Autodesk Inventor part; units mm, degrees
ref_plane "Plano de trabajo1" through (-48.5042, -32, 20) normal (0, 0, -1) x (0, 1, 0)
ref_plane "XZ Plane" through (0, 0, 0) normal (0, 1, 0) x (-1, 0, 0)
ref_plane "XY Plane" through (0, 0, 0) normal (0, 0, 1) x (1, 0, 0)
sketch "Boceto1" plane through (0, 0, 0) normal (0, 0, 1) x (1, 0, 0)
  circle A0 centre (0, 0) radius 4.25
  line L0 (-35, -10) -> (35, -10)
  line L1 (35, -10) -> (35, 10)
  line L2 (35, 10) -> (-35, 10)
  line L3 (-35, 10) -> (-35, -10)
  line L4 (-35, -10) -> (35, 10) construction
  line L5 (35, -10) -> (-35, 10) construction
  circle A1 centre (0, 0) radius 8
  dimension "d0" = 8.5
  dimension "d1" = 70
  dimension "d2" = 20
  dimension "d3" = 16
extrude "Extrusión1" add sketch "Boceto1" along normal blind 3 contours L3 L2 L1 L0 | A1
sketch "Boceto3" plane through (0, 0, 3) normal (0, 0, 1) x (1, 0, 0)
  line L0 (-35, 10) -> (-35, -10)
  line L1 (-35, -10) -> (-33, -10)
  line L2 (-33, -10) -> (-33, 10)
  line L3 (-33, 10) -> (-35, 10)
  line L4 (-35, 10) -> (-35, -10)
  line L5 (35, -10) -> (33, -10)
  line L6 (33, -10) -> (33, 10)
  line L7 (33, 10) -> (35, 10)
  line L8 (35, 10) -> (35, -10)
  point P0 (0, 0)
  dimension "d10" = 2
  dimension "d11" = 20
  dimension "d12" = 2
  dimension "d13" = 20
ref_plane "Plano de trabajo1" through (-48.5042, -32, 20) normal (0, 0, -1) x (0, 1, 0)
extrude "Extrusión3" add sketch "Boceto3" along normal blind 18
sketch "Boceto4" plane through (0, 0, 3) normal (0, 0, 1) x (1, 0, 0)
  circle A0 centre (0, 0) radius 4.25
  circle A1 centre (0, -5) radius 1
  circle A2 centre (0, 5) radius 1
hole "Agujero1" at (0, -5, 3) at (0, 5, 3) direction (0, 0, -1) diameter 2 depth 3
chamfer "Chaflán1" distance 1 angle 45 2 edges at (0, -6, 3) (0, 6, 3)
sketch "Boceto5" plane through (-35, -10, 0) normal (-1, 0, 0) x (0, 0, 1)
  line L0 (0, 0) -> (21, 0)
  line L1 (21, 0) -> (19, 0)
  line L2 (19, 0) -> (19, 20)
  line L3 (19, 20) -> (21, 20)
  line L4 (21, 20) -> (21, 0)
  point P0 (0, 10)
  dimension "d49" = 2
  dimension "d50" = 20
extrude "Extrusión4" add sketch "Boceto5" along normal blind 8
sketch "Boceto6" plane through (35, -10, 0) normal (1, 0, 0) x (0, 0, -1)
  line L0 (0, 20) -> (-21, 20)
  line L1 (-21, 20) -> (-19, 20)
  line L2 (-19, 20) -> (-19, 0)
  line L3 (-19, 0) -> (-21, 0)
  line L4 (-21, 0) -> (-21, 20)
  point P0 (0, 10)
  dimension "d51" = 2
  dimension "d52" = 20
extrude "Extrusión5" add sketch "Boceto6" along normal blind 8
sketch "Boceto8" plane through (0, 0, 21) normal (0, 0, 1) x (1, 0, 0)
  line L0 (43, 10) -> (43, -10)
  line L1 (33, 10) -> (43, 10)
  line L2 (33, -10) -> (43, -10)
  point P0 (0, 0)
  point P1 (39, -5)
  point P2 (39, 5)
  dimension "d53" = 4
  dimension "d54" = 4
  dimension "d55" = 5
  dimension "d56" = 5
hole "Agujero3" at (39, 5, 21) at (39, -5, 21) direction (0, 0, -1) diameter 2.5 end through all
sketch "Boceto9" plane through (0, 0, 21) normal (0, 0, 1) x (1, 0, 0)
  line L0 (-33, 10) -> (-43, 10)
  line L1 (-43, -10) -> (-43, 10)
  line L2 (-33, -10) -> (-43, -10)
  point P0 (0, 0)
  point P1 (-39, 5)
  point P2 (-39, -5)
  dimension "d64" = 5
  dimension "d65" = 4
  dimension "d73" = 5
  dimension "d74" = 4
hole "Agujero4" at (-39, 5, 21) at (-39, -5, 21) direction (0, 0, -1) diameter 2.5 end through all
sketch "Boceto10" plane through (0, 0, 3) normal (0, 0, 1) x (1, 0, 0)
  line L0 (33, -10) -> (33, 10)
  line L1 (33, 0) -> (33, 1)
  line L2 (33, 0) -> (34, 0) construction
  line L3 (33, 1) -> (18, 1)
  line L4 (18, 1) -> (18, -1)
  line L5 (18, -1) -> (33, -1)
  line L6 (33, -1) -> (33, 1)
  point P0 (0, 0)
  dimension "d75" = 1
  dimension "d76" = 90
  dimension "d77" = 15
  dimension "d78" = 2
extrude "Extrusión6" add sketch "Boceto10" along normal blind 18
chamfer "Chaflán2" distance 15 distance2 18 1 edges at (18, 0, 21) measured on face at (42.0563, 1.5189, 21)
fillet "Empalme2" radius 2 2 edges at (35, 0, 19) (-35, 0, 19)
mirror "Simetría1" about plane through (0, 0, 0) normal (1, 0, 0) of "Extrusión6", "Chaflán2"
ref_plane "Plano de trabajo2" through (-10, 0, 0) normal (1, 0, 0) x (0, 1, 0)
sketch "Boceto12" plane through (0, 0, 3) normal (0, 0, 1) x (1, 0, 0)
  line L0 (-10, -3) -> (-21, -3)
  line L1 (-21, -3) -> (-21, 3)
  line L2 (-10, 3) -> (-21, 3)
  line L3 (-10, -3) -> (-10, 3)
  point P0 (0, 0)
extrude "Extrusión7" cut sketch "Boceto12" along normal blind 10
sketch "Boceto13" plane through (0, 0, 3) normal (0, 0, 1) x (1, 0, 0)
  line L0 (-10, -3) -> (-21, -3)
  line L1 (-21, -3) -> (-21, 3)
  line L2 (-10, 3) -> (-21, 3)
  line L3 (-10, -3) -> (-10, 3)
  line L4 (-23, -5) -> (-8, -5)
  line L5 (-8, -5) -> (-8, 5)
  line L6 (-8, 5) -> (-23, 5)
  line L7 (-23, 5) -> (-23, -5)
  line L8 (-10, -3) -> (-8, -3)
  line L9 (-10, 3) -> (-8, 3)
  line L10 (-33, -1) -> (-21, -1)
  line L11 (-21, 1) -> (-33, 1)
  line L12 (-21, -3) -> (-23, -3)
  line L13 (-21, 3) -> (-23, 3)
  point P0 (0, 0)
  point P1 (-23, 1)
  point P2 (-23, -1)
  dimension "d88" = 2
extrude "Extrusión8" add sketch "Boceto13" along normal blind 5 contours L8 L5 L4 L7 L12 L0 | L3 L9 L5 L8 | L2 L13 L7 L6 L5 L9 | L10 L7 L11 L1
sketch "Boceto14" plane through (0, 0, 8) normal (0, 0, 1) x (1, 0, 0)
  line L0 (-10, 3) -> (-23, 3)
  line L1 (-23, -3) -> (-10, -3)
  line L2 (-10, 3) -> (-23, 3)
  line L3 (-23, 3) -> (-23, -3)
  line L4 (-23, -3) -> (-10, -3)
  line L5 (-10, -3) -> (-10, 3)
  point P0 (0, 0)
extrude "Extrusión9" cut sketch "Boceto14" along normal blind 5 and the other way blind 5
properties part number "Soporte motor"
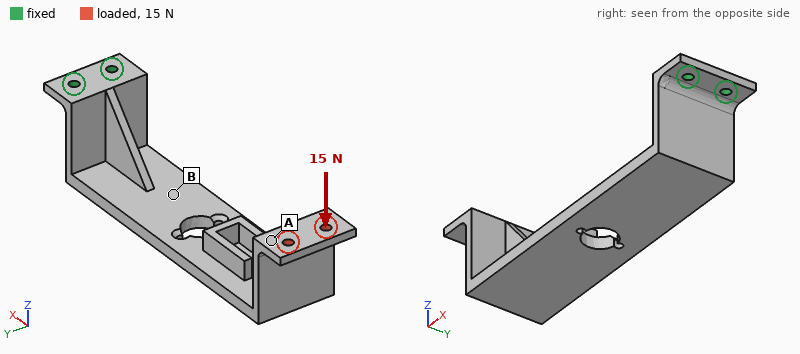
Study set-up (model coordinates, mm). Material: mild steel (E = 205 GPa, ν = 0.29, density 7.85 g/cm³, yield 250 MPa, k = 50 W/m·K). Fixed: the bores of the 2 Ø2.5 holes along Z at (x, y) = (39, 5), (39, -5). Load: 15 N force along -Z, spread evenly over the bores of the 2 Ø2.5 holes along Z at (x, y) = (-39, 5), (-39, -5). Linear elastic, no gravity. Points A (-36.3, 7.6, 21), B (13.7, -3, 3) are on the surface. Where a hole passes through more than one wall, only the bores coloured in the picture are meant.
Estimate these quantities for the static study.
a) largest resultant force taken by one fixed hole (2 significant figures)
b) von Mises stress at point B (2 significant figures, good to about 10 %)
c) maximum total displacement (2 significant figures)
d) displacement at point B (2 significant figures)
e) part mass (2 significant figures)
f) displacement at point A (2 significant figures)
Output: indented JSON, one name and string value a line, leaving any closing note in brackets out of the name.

{
  "largest resultant force taken by one fixed hole": "13 N",
  "von Mises stress at point B": "25 MPa",
  "maximum total displacement": "0.36 mm",
  "displacement at point B": "0.069 mm",
  "part mass": "55 g",
  "displacement at point A": "0.33 mm"
}
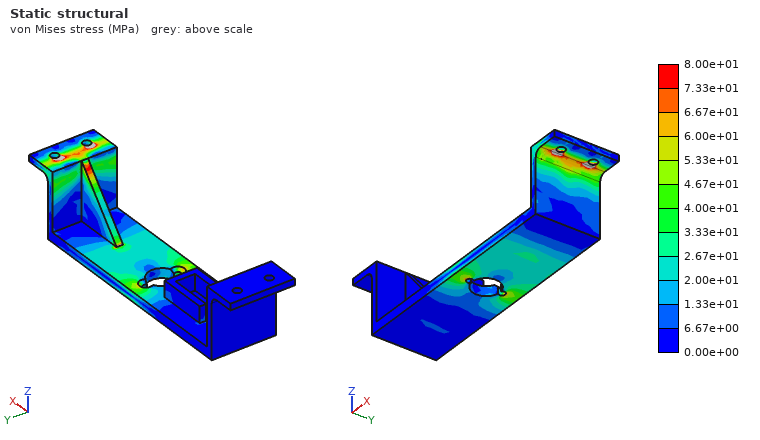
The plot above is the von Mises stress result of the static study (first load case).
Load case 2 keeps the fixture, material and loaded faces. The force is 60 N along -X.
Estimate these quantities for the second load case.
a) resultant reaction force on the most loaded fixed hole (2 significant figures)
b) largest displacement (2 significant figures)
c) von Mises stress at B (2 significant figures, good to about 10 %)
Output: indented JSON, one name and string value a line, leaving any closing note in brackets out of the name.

{
  "resultant reaction force on the most loaded fixed hole": "33 N",
  "largest displacement": "0.32 mm",
  "von Mises stress at B": "36 MPa"
}
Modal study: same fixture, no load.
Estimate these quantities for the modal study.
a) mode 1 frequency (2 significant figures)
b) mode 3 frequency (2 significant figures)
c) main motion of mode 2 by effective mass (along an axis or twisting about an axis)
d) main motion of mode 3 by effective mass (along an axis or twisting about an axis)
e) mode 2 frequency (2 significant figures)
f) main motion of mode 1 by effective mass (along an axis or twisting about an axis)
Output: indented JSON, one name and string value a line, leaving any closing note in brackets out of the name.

{
  "mode 1 frequency": "250 Hz",
  "mode 3 frequency": "1000 Hz",
  "main motion of mode 2 by effective mass": "along Y",
  "main motion of mode 3 by effective mass": "along X",
  "mode 2 frequency": "350 Hz",
  "main motion of mode 1 by effective mass": "along Z"
}
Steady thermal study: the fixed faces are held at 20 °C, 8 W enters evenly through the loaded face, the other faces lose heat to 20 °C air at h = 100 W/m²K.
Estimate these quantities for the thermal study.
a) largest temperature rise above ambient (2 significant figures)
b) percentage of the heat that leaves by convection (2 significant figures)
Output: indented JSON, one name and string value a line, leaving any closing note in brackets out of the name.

{
  "largest temperature rise above ambient": "65 K",
  "percentage of the heat that leaves by convection": "99 %"
}
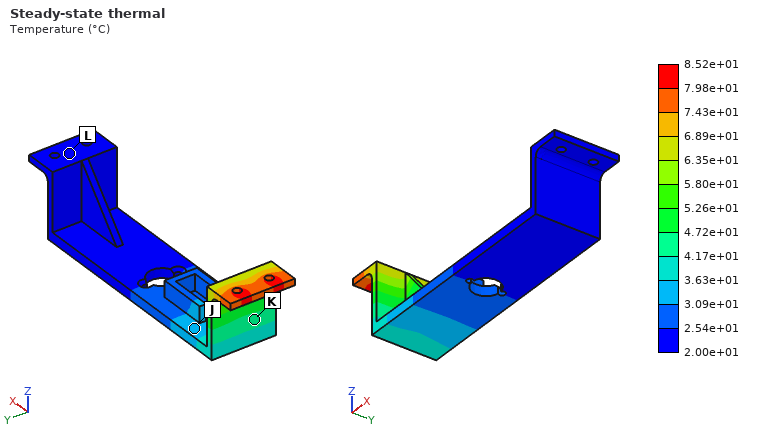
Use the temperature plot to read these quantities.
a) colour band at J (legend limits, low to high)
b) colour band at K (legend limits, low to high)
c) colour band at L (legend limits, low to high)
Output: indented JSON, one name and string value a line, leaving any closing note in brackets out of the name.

{
  "colour band at J": "3.09e+01 to 3.63e+01 °C",
  "colour band at K": "4.17e+01 to 4.72e+01 °C",
  "colour band at L": "2.00e+01 to 2.54e+01 °C"
}
